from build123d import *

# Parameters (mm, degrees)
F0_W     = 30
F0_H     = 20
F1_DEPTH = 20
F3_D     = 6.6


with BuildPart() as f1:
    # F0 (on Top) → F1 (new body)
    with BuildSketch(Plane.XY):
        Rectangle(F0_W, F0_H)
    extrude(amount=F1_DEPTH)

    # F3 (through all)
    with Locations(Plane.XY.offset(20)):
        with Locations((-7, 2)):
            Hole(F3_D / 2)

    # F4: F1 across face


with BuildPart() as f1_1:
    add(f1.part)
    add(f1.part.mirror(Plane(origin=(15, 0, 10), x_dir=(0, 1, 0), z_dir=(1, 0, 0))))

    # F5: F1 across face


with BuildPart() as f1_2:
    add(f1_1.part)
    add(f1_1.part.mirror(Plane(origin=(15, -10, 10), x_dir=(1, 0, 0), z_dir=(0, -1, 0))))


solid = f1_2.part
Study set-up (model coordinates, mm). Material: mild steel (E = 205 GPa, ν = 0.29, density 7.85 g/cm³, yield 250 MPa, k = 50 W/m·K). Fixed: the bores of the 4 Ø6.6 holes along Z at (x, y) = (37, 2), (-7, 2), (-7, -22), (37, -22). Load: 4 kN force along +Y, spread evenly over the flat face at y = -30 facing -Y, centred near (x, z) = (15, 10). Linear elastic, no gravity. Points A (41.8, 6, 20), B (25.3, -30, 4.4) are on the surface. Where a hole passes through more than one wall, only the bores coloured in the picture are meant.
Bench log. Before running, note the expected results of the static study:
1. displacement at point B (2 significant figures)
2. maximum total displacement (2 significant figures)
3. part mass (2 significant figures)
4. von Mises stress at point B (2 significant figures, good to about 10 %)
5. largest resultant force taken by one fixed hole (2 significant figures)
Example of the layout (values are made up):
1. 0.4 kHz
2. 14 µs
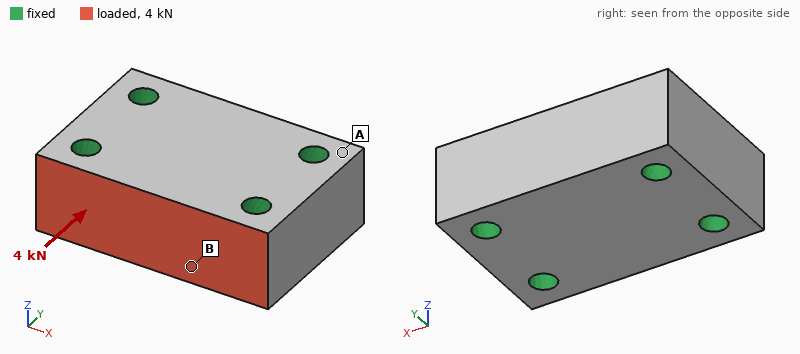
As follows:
1. 0.40 µm
2. 0.51 µm
3. 360 g
4. 2.9 MPa
5. 1.5 kN
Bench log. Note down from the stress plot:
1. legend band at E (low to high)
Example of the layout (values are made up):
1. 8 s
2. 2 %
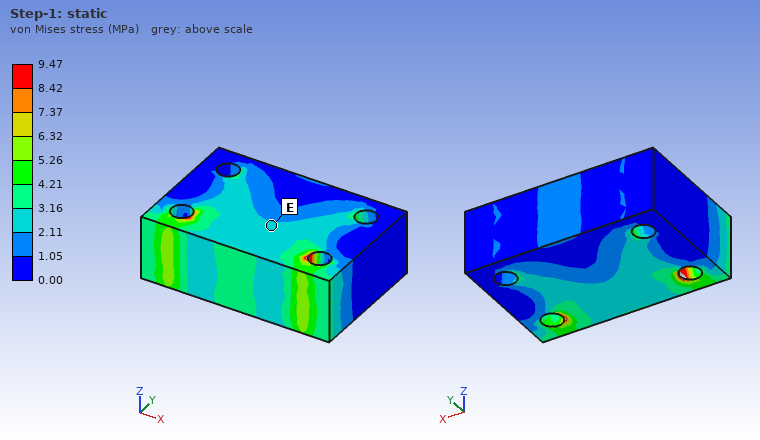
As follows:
1. 2.11 to 3.16 MPa
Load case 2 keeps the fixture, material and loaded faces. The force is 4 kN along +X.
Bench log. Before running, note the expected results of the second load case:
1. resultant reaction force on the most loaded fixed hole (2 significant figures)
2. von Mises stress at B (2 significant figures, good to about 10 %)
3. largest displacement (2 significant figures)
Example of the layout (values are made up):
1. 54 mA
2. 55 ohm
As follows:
1. 1.9 kN
2. 6.1 MPa
3. 0.63 µm
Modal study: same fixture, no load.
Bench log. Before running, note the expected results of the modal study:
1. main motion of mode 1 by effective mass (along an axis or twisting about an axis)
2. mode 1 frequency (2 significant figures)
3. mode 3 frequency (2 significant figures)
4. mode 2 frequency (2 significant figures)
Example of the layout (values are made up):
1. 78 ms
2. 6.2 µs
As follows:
1. along Z
2. 29 kHz
3. 34 kHz
4. 34 kHz
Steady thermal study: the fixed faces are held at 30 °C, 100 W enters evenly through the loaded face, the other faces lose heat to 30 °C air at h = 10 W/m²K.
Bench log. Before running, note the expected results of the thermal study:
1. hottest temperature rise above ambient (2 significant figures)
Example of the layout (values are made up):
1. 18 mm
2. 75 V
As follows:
1. 27 K
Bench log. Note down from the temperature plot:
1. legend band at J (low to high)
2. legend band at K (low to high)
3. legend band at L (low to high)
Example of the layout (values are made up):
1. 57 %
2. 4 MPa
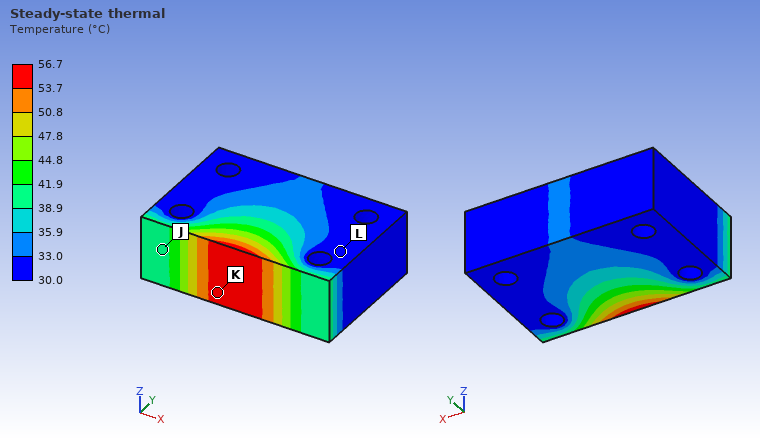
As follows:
1. 38.9 to 41.9 °C
2. 53.7 to 56.7 °C
3. 30.0 to 33.0 °C
